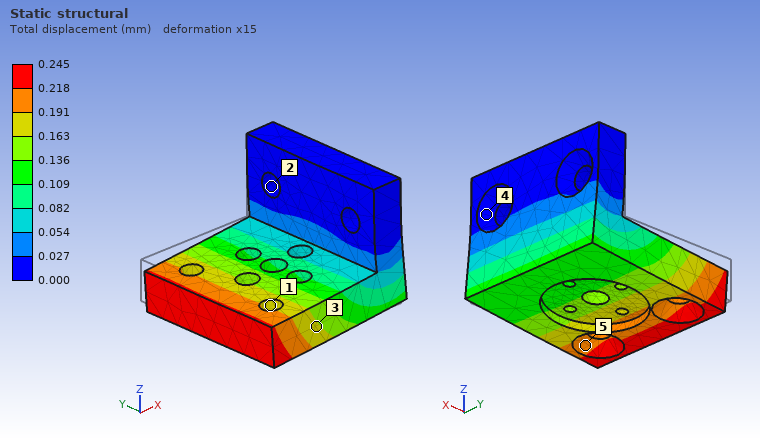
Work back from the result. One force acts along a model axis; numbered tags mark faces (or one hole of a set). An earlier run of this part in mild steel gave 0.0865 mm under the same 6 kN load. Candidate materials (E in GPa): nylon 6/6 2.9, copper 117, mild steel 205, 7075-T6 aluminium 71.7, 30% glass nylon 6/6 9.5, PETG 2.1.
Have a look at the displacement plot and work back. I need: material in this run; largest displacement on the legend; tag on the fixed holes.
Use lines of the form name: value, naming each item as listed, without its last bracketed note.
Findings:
material in this run: 7075-T6 aluminium
largest displacement on the legend: 0.245 mm
tag on the fixed holes: 2
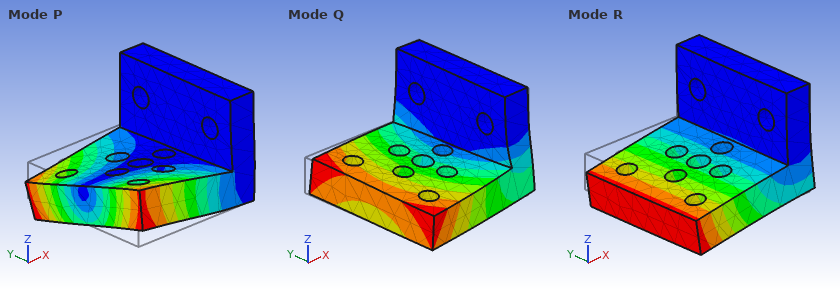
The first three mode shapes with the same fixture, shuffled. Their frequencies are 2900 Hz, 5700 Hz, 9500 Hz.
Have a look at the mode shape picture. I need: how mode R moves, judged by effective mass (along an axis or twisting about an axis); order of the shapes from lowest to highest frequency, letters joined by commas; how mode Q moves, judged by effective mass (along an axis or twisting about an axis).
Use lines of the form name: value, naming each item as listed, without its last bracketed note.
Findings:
how mode R moves, judged by effective mass: along Z
order of the shapes from lowest to highest frequency, letters joined by commas: R, Q, P
how mode Q moves, judged by effective mass: along Y
